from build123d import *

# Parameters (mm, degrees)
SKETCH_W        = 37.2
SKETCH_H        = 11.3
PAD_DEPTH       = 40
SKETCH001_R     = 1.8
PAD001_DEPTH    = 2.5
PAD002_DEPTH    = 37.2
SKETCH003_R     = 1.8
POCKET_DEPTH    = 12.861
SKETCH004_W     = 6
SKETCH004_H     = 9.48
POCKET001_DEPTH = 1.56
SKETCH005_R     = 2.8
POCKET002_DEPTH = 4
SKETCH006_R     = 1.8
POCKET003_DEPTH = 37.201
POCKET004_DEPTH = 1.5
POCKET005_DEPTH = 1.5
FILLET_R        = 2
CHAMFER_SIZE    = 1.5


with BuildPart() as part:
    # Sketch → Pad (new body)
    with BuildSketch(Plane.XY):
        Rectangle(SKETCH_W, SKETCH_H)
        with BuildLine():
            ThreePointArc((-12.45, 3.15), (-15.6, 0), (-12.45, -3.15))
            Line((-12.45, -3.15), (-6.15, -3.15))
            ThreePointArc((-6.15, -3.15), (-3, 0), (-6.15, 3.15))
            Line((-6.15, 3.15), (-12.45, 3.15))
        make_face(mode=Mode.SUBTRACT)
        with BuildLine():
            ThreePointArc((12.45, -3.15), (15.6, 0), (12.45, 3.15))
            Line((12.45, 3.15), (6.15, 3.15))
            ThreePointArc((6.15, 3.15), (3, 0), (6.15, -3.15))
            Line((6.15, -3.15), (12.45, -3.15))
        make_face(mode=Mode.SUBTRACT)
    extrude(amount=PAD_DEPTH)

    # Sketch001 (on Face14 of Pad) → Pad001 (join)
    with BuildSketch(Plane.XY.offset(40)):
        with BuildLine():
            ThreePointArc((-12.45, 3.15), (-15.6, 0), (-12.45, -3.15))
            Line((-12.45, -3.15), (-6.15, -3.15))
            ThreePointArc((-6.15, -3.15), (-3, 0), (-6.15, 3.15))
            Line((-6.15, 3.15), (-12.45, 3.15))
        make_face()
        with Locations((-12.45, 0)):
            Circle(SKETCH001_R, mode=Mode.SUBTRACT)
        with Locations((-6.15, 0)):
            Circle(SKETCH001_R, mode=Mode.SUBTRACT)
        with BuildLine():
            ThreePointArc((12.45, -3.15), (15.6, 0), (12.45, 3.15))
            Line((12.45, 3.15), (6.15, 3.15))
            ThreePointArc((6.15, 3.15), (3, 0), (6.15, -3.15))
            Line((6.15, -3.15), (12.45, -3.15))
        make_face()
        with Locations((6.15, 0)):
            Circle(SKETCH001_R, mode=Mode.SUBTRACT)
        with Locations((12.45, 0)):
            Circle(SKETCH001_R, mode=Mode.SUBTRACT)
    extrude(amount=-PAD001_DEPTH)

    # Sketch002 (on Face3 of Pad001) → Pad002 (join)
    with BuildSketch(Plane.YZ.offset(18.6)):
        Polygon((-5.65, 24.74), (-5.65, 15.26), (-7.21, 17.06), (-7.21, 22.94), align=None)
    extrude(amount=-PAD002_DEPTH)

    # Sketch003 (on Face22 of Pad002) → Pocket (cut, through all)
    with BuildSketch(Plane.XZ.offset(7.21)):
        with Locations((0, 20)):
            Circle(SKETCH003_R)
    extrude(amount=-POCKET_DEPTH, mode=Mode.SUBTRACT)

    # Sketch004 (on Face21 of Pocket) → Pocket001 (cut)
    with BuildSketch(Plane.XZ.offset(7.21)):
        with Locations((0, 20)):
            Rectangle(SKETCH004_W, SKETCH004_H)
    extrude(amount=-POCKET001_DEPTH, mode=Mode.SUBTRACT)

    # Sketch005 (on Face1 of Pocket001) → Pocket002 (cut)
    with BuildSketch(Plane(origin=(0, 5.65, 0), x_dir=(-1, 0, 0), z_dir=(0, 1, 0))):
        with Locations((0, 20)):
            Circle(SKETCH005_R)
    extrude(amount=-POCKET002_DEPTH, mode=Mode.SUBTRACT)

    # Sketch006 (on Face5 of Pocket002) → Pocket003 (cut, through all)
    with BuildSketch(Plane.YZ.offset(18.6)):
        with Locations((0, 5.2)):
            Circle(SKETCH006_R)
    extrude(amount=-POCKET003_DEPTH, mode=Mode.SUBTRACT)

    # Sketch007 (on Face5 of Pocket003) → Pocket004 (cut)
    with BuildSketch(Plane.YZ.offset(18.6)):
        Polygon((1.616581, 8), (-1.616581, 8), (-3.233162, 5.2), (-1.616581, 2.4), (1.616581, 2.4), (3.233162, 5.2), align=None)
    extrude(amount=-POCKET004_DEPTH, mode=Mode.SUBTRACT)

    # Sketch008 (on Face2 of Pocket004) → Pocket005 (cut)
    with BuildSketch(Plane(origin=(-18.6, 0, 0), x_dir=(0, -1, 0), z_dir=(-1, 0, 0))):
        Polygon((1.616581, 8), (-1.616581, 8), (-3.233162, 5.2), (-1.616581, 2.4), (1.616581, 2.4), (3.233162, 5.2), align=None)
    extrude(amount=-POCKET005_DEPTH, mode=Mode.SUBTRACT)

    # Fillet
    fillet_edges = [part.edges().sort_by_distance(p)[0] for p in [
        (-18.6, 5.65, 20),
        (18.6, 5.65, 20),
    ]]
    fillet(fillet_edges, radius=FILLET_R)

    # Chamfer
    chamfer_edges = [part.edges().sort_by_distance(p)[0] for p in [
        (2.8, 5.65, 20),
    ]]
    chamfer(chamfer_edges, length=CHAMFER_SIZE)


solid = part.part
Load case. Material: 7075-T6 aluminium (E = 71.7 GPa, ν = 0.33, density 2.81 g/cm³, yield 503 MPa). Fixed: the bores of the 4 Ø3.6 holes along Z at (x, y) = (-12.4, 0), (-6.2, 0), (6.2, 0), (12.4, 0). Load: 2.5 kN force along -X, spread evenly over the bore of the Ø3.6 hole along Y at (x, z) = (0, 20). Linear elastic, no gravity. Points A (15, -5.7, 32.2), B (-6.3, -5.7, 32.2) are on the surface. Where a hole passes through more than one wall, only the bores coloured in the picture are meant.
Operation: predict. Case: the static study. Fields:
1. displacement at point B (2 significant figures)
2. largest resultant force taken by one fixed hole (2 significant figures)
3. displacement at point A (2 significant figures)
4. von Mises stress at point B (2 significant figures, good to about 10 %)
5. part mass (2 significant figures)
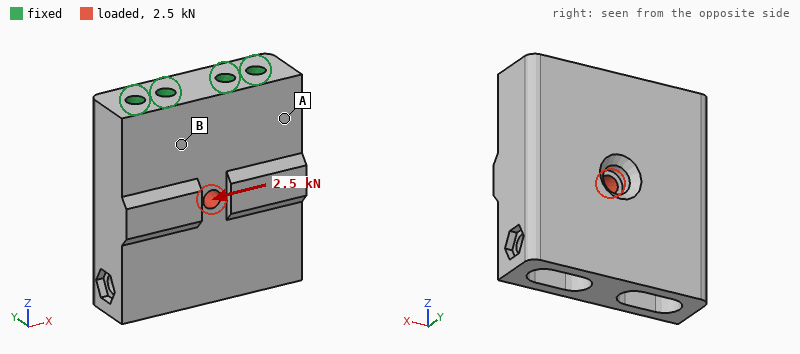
9.0 µm
1.5 kN
13 µm
38 MPa
32 g
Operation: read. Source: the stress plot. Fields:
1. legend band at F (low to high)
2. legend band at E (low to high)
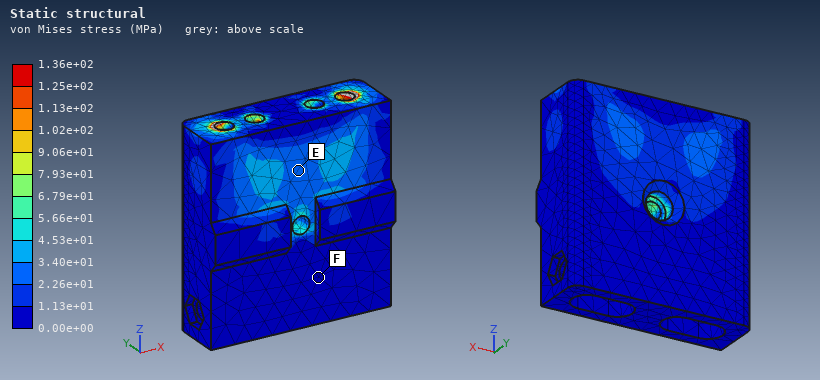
0.00e+00 to 1.13e+01 MPa
2.26e+01 to 3.40e+01 MPa
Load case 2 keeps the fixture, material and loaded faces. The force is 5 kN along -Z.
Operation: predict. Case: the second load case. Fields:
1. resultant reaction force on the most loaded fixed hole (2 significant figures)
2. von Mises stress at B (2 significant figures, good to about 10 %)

1.4 kN
43 MPa
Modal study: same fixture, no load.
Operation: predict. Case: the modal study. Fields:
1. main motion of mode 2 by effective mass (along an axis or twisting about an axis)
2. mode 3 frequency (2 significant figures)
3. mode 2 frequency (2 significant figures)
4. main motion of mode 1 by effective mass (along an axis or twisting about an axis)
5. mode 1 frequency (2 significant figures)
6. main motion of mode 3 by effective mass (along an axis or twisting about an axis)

along X
10 kHz
8500 Hz
along Y
3000 Hz
twisting about Z
